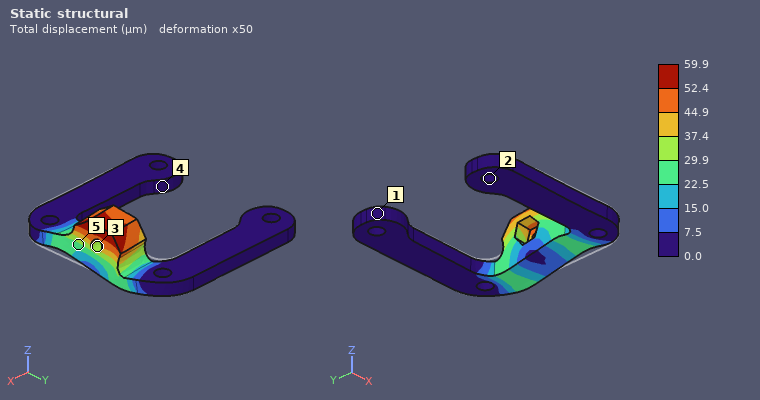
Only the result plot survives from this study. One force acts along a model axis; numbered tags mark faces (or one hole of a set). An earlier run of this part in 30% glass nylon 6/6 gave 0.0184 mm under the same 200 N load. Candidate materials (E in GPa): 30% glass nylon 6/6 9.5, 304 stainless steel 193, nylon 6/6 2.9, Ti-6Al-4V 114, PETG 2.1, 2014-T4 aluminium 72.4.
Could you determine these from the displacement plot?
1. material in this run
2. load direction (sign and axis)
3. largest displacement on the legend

nylon 6/6
+Y
59.9 µm
